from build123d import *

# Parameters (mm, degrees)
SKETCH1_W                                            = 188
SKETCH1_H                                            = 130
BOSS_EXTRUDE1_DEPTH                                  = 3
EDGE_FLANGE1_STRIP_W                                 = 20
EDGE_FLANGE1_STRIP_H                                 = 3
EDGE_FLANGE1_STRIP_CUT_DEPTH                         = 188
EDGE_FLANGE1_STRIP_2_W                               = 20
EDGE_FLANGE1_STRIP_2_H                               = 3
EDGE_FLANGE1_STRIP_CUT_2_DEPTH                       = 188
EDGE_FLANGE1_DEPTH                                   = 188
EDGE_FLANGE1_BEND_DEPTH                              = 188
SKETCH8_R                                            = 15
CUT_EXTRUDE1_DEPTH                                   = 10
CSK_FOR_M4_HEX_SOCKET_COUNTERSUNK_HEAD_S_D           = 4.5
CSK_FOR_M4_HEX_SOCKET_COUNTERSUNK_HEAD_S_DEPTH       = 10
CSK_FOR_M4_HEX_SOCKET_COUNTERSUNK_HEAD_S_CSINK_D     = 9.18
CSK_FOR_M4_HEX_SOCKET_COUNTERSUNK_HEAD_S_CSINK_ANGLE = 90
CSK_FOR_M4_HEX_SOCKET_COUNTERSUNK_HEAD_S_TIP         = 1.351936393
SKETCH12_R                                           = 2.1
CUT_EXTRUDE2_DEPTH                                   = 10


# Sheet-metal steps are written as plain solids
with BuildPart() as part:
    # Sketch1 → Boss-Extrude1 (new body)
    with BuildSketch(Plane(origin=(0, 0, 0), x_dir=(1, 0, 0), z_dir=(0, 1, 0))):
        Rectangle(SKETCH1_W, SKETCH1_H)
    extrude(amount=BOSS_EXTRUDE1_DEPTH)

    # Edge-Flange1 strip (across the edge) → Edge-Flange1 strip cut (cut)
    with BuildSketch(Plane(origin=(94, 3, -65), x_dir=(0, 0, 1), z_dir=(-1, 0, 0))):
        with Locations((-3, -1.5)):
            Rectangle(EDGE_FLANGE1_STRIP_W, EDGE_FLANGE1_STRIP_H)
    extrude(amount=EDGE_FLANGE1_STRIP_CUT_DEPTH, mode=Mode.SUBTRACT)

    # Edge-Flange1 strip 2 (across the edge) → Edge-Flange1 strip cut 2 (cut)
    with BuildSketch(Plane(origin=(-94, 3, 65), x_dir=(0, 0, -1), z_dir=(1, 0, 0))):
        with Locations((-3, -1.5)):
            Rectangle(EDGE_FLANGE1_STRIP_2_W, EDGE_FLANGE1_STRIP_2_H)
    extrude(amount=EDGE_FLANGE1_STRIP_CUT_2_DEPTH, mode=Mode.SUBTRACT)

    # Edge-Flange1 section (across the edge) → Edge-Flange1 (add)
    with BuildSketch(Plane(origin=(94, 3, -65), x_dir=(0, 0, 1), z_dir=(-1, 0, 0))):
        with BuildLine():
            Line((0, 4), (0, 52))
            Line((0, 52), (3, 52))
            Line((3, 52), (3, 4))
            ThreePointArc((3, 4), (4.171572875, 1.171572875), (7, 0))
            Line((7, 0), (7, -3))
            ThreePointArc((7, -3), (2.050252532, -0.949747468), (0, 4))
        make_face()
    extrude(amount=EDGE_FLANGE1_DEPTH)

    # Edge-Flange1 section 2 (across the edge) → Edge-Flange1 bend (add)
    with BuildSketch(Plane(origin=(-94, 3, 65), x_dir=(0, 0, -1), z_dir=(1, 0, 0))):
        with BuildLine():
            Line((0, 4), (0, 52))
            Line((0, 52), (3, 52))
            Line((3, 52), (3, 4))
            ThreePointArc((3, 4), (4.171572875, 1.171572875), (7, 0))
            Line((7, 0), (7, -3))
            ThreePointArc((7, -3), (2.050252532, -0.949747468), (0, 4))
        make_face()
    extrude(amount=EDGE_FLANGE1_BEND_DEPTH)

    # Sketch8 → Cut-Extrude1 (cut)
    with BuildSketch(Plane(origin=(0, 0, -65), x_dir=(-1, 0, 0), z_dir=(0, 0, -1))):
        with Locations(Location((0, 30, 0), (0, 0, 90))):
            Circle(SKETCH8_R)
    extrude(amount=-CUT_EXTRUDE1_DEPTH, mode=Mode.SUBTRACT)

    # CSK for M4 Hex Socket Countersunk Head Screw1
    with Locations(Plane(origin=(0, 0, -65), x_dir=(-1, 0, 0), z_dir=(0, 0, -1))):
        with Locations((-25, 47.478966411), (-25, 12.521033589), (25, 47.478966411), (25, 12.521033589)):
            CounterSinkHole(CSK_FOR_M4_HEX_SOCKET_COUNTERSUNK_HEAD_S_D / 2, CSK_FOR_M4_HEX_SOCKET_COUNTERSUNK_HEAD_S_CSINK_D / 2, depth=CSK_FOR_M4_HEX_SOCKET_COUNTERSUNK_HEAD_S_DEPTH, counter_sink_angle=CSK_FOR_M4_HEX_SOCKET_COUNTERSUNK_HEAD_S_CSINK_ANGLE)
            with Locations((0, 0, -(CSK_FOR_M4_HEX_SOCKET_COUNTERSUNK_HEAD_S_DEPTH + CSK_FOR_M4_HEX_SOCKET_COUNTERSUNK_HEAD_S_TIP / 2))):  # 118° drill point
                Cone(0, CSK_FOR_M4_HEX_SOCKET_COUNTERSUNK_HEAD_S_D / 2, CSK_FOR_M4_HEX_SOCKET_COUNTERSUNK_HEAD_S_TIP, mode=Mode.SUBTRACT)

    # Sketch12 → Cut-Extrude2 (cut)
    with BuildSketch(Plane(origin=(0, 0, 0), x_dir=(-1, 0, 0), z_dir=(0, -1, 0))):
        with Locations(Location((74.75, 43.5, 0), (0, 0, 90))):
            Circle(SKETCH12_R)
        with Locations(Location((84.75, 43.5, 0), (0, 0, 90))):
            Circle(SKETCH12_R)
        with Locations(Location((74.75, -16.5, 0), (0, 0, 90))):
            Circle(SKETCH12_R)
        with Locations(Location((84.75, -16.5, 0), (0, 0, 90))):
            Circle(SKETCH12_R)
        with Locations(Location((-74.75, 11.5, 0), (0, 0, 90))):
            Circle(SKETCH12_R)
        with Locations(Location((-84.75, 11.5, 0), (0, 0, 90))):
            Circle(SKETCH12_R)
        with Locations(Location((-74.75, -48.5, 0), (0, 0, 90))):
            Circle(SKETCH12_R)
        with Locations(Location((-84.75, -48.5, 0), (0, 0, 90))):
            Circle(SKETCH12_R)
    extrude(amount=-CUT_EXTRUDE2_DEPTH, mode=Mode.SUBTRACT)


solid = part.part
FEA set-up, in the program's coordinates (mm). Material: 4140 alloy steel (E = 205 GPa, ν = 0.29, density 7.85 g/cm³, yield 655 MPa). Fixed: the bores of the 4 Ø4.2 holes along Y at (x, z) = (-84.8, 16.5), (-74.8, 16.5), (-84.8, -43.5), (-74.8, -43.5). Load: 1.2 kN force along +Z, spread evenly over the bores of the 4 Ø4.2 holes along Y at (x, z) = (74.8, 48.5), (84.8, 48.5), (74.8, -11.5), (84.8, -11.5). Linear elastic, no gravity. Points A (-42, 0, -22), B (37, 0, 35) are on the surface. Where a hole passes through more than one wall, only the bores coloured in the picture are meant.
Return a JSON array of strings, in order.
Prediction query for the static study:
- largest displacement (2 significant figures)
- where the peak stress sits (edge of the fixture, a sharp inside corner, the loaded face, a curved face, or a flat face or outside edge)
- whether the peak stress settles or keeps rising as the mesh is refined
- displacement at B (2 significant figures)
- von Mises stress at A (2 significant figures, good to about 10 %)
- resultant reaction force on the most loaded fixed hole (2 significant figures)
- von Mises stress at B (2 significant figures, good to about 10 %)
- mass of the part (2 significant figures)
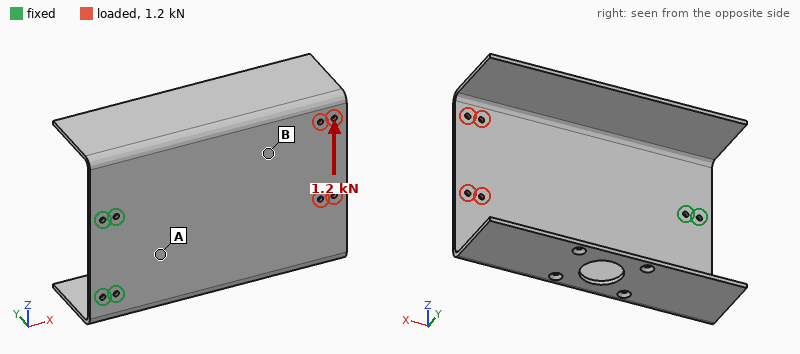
["48 µm", "edge of the fixture", "keeps rising", "29 µm", "16 MPa", "2.2 kN", "5.2 MPa", "990 g"]
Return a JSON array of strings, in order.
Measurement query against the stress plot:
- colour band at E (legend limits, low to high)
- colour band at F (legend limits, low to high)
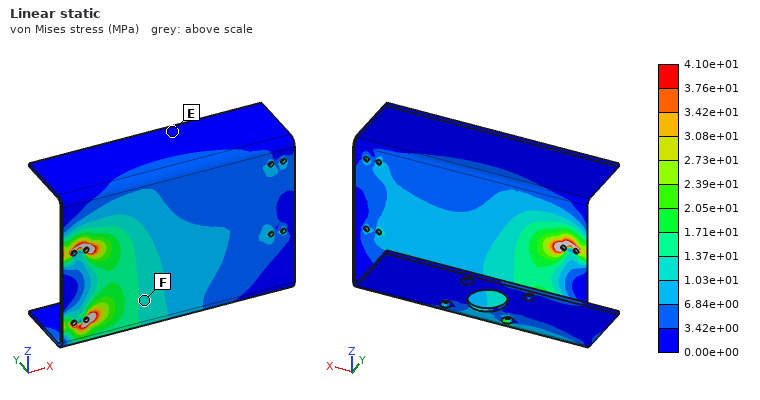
["0.00e+00 to 3.42e+00 MPa", "1.03e+01 to 1.37e+01 MPa"]
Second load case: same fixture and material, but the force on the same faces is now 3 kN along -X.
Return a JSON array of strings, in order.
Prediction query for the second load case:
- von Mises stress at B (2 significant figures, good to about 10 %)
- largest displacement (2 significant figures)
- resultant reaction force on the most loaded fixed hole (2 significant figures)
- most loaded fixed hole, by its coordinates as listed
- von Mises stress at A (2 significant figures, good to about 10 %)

["10.0 MPa", "25 µm", "2.0 kN", "(-74.8, 16.5)", "6.6 MPa"]
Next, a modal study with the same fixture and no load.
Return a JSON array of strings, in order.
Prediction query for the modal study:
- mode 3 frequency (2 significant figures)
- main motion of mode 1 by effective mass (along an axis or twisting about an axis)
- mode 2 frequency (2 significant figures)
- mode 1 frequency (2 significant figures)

["350 Hz", "along Y", "160 Hz", "100 Hz"]
